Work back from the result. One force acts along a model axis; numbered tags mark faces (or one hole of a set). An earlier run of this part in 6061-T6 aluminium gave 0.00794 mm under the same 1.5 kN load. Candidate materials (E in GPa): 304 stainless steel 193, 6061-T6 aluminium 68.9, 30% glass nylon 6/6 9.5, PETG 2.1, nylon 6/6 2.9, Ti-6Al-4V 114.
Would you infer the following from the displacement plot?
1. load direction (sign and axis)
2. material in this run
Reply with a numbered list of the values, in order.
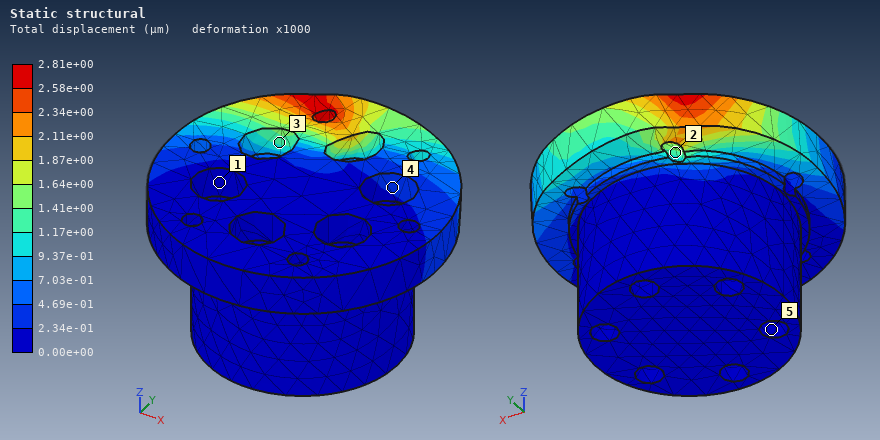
1. +X
2. 304 stainless steel
